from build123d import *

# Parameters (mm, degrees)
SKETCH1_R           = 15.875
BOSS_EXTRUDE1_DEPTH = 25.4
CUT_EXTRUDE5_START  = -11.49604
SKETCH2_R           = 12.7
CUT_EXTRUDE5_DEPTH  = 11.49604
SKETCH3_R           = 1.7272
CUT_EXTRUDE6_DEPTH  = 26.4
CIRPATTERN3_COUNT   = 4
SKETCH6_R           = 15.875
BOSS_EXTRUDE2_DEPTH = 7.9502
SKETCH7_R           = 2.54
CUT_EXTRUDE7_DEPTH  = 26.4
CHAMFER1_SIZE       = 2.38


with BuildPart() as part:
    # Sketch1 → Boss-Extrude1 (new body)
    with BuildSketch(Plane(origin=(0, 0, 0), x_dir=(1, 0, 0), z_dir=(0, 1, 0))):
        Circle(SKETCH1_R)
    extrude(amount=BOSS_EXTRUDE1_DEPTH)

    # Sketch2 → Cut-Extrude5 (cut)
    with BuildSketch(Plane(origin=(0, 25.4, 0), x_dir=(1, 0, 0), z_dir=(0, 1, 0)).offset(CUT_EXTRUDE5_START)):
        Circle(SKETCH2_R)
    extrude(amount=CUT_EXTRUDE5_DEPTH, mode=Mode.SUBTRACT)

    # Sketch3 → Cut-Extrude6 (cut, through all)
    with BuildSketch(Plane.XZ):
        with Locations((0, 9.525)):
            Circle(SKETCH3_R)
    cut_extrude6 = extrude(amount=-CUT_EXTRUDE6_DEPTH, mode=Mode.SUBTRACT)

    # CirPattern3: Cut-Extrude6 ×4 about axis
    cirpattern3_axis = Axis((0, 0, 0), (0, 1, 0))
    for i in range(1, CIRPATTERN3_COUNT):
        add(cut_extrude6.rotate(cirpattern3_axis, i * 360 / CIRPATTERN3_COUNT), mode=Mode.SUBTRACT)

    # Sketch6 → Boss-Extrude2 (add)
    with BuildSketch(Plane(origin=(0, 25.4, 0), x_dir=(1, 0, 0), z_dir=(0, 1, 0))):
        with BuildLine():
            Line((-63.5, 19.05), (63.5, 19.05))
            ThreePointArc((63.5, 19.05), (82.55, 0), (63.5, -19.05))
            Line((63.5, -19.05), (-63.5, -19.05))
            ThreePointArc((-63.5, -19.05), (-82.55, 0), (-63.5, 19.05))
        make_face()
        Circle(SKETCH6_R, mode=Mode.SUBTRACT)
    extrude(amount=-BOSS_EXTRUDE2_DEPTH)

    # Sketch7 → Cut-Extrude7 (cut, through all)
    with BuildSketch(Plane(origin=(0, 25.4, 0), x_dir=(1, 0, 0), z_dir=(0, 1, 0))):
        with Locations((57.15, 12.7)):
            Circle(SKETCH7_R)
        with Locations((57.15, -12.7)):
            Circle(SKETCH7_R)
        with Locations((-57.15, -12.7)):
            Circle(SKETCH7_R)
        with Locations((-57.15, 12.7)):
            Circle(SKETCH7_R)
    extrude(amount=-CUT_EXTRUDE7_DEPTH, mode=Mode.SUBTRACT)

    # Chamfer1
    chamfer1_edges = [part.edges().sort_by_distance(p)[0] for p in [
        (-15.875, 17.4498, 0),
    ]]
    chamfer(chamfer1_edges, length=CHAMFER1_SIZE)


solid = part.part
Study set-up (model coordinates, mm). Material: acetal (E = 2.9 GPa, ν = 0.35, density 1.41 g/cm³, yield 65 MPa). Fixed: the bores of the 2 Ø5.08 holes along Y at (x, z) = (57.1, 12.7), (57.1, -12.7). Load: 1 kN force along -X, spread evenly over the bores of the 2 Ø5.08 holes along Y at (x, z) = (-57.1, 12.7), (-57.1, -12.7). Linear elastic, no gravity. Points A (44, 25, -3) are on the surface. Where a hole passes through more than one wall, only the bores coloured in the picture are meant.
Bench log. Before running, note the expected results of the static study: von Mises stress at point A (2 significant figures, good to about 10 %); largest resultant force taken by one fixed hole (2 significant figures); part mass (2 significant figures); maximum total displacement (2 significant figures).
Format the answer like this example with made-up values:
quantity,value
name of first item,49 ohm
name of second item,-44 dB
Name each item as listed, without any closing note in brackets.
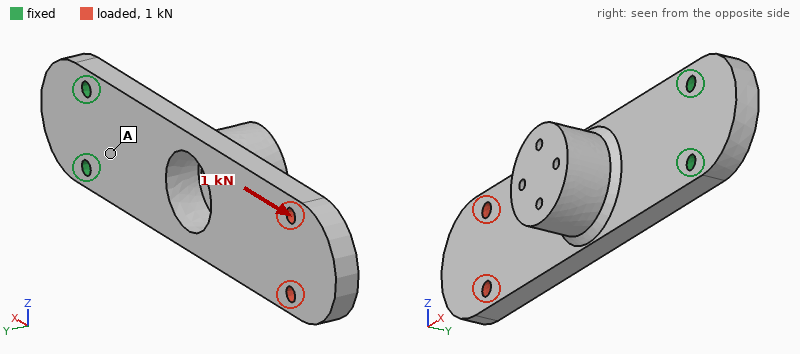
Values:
quantity,value
von Mises stress at point A,2.6 MPa
largest resultant force taken by one fixed hole,500 N
part mass,77 g
maximum total displacement,0.77 mm
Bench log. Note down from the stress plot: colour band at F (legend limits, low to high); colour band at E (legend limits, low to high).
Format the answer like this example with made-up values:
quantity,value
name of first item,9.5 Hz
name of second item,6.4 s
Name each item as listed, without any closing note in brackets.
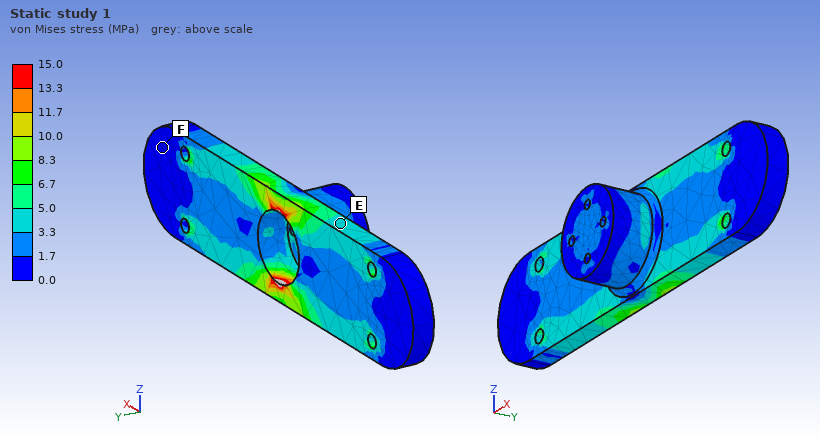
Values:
quantity,value
colour band at F,0.0 to 1.7 MPa
colour band at E,3.3 to 5.0 MPa
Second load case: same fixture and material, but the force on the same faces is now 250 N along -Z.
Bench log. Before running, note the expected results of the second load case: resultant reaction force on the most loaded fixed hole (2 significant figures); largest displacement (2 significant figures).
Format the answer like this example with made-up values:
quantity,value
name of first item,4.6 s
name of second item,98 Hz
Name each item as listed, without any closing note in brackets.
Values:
quantity,value
resultant reaction force on the most loaded fixed hole,1.1 kN
largest displacement,1.9 mm
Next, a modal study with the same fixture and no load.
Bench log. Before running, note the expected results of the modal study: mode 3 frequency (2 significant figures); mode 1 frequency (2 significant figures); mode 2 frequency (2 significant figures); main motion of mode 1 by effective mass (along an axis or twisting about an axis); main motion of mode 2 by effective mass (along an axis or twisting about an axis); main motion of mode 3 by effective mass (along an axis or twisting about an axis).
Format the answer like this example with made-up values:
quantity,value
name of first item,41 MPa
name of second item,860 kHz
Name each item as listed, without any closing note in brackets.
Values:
quantity,value
mode 3 frequency,600 Hz
mode 1 frequency,100 Hz
mode 2 frequency,420 Hz
main motion of mode 1 by effective mass,along Y
main motion of mode 2 by effective mass,along Z
main motion of mode 3 by effective mass,along Y
